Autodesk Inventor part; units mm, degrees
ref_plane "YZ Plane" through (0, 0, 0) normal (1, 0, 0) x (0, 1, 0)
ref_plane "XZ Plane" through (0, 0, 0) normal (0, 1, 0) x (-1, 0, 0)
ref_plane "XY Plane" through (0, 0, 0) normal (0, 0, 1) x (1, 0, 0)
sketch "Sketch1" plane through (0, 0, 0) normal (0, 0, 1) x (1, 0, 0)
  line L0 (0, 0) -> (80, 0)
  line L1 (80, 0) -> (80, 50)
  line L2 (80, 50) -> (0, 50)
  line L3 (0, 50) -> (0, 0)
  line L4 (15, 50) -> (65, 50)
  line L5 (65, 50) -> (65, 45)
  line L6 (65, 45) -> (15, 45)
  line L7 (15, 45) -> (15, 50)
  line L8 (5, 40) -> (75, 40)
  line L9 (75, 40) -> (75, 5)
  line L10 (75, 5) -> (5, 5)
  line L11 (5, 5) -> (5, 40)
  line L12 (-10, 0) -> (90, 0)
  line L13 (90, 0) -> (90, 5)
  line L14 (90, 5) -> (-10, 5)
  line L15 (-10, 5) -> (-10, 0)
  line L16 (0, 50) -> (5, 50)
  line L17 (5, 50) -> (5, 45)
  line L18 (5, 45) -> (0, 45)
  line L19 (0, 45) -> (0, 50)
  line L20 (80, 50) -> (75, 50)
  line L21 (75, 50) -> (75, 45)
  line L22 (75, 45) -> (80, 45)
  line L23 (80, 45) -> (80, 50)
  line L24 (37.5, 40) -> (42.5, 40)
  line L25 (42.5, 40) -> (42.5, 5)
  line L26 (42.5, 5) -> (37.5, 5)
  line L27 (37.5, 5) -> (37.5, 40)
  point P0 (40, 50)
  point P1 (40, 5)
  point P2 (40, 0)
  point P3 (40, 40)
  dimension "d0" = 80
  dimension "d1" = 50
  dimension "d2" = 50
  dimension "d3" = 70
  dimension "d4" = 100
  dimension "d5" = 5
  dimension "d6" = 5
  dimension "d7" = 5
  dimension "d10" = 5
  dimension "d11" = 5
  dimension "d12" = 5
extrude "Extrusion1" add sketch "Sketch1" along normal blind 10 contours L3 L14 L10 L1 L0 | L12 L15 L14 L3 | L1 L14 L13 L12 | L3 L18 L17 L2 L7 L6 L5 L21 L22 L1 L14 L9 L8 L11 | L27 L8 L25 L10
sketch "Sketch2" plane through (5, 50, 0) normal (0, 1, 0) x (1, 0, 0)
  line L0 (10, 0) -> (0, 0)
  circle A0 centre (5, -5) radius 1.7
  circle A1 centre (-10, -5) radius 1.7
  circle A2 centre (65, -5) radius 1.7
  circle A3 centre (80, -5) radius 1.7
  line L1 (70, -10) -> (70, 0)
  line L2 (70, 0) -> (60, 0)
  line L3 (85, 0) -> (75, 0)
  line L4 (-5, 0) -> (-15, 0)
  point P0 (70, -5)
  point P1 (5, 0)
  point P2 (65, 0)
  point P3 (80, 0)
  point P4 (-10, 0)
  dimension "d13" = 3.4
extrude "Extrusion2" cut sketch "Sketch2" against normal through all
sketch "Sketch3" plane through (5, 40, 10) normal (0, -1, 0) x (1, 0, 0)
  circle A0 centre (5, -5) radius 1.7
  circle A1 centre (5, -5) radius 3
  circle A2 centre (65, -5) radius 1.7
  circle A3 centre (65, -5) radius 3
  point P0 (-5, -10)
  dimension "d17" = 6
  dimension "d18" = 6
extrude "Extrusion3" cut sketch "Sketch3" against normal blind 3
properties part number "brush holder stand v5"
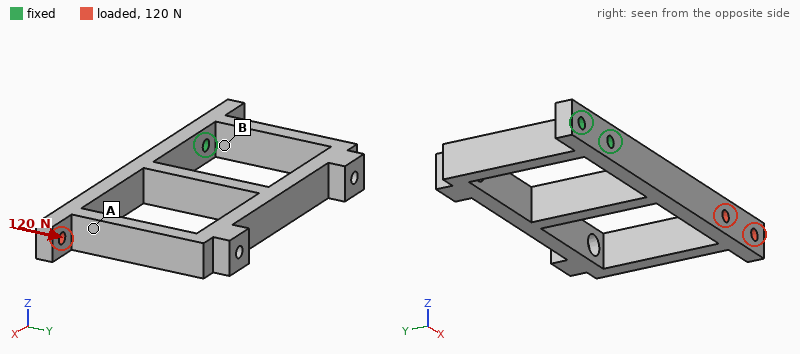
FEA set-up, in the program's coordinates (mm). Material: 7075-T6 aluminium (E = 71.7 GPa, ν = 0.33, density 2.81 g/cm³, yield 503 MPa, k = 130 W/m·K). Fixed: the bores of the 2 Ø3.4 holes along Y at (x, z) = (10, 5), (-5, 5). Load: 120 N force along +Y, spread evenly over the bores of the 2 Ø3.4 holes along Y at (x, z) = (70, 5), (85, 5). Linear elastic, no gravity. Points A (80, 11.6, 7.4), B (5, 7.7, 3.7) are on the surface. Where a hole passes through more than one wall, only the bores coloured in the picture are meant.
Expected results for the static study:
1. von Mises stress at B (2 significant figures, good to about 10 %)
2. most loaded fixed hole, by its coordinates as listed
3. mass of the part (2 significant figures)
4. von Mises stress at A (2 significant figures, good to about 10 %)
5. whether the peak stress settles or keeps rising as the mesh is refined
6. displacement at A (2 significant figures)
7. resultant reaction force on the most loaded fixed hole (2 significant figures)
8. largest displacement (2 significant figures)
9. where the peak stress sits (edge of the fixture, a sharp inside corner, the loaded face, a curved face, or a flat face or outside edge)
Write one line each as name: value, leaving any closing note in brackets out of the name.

von Mises stress at B: 60 MPa
most loaded fixed hole, by its coordinates as listed: (10, 5)
mass of the part: 42 g
von Mises stress at A: 13 MPa
whether the peak stress settles or keeps rising as the mesh is refined: keeps rising
displacement at A: 0.39 mm
resultant reaction force on the most loaded fixed hole: 480 N
largest displacement: 0.44 mm
where the peak stress sits: edge of the fixture
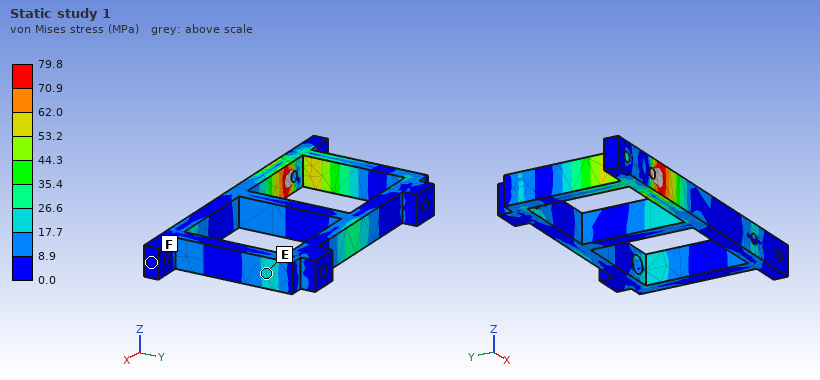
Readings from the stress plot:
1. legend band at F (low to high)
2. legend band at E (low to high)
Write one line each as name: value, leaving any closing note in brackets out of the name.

legend band at F: 0.0 to 8.9 MPa
legend band at E: 17.7 to 26.6 MPa
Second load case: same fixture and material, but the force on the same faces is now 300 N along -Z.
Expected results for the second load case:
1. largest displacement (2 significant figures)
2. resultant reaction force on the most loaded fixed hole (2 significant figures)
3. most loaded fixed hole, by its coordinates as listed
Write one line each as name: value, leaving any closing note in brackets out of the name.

largest displacement: 1.2 mm
resultant reaction force on the most loaded fixed hole: 990 N
most loaded fixed hole, by its coordinates as listed: (10, 5)
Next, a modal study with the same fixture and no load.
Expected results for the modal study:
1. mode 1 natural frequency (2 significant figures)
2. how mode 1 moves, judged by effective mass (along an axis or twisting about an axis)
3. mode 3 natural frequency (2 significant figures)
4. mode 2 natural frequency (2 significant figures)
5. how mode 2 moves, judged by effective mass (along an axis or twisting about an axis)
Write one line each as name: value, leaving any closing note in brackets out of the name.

mode 1 natural frequency: 620 Hz
how mode 1 moves, judged by effective mass: along Z
mode 3 natural frequency: 1400 Hz
mode 2 natural frequency: 650 Hz
how mode 2 moves, judged by effective mass: along Y
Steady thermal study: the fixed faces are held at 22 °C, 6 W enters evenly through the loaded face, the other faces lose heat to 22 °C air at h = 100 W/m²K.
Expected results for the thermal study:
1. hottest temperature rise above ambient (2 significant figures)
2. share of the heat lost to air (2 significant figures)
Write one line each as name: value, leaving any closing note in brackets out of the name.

hottest temperature rise above ambient: 19 K
share of the heat lost to air: 79 %
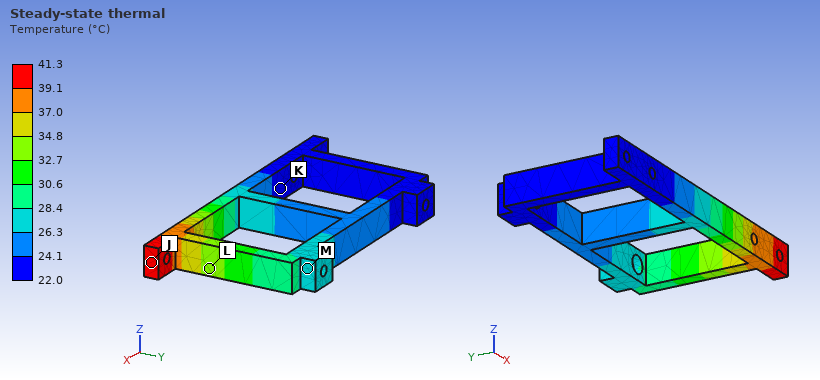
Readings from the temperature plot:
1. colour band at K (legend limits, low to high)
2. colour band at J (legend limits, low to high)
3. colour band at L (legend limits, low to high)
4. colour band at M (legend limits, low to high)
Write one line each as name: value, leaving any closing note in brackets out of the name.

colour band at K: 22.0 to 24.1 °C
colour band at J: 39.1 to 41.3 °C
colour band at L: 32.7 to 34.8 °C
colour band at M: 26.3 to 28.4 °C
